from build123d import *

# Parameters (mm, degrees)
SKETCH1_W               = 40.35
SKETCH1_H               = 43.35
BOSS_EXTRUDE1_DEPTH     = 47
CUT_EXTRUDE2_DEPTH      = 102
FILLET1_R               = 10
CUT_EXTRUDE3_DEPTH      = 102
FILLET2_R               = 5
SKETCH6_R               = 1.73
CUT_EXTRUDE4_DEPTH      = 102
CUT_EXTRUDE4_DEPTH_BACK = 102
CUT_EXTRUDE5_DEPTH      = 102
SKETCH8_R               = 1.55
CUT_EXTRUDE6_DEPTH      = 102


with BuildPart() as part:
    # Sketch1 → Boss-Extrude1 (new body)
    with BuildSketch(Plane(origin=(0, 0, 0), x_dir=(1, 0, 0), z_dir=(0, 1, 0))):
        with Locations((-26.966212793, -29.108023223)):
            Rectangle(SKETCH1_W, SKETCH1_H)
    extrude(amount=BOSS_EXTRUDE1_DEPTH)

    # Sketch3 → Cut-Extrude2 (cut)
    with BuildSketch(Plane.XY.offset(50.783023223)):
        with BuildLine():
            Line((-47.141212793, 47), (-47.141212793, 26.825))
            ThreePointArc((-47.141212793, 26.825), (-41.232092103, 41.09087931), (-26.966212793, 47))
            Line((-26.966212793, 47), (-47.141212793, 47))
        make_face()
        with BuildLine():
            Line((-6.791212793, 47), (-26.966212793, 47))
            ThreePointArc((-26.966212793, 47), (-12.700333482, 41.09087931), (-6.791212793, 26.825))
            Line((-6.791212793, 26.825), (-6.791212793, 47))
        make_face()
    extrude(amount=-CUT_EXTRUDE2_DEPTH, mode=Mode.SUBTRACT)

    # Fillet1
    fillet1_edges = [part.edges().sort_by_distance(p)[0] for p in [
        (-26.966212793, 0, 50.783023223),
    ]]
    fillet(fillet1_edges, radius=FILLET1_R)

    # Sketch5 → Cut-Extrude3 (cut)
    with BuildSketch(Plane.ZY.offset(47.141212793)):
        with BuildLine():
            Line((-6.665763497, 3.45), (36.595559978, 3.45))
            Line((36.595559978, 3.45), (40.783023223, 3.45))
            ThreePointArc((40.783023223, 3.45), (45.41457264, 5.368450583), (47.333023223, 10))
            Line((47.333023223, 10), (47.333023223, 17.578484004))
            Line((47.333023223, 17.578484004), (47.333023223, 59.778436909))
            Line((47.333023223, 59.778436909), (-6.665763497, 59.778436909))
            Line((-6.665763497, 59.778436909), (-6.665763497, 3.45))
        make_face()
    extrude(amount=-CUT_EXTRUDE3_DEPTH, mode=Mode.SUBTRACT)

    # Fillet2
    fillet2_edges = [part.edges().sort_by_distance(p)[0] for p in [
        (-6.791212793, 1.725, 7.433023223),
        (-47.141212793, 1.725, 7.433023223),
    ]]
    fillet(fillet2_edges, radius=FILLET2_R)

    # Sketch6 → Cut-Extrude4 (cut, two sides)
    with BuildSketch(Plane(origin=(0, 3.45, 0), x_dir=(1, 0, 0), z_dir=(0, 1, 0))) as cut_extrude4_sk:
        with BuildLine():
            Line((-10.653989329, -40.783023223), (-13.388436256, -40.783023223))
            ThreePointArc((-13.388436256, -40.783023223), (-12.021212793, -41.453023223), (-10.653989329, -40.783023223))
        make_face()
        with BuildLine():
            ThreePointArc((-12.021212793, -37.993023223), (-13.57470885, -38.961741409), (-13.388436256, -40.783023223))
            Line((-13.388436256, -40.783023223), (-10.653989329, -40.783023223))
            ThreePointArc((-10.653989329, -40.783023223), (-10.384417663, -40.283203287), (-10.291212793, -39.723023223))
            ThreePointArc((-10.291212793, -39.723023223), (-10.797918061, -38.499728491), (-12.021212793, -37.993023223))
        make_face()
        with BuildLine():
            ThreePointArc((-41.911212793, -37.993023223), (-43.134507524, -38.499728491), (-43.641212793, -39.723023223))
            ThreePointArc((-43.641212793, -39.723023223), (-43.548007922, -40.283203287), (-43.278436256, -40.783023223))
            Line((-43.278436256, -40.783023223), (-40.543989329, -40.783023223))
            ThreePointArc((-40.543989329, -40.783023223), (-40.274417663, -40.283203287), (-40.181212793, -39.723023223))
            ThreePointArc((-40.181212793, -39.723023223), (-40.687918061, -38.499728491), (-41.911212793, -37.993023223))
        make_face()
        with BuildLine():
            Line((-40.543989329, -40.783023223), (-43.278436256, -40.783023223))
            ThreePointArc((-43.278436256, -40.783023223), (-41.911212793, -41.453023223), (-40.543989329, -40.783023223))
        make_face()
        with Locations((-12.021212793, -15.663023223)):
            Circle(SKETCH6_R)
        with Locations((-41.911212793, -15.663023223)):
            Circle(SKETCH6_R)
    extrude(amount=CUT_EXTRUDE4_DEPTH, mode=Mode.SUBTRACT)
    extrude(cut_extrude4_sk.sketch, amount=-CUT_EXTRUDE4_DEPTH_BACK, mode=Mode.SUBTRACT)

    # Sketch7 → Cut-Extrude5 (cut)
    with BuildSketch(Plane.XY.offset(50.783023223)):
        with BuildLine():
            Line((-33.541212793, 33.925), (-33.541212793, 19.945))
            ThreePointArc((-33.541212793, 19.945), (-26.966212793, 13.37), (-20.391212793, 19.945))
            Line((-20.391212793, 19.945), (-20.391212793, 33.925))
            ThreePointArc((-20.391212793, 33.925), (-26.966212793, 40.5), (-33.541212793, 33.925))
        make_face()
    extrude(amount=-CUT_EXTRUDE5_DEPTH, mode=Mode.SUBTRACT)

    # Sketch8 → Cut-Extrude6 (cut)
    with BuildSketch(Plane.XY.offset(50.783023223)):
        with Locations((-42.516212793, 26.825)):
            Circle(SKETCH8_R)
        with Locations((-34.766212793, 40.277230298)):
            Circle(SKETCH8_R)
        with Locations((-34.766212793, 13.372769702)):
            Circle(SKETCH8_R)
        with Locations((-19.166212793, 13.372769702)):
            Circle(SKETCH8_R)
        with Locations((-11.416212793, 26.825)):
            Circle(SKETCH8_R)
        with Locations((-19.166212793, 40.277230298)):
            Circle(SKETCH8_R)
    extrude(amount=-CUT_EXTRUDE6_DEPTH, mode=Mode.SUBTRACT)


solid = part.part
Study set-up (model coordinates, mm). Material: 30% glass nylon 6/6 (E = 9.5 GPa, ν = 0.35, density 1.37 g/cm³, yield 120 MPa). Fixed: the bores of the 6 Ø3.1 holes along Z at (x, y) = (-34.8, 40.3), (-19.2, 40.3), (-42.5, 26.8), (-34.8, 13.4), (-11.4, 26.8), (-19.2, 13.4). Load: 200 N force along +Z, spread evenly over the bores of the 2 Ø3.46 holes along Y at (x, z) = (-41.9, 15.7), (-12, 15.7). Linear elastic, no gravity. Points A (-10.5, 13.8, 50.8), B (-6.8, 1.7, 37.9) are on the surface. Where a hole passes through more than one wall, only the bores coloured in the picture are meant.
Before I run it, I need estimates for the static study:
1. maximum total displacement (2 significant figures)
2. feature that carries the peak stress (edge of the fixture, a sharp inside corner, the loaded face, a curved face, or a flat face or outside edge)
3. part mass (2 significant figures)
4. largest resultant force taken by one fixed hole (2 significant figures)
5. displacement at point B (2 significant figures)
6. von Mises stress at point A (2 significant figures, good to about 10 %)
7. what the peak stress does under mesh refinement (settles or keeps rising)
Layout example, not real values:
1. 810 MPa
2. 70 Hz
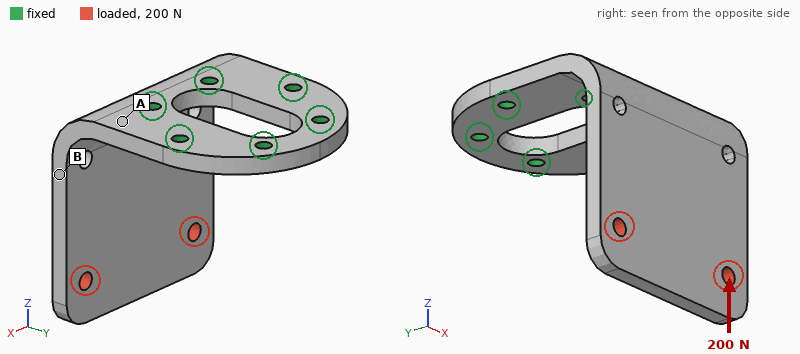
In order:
1. 0.51 mm
2. edge of the fixture
3. 13 g
4. 120 N
5. 0.16 mm
6. 11 MPa
7. keeps rising
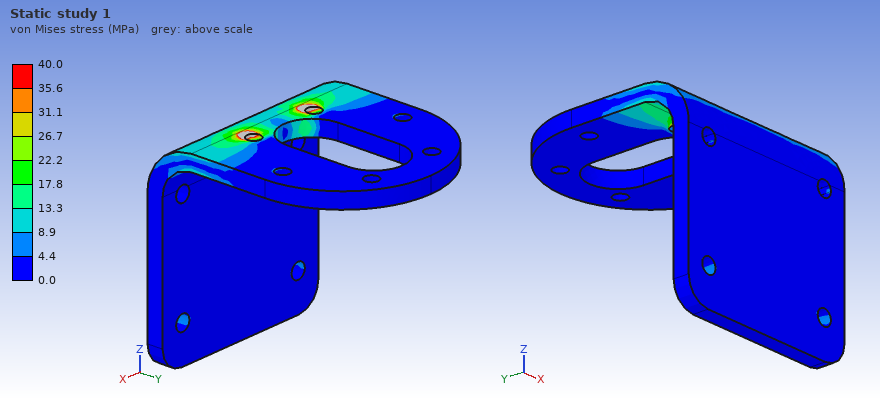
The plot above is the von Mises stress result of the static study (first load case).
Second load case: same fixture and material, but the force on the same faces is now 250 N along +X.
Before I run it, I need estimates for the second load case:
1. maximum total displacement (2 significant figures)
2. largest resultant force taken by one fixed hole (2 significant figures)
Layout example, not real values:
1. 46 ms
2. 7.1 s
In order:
1. 0.83 mm
2. 460 N
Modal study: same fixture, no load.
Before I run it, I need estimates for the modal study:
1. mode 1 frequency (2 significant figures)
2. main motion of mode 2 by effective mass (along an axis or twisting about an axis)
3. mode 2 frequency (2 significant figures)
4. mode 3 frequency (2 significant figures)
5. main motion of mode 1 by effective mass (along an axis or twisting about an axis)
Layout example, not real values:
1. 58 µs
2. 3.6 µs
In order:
1. 640 Hz
2. along X
3. 1400 Hz
4. 2300 Hz
5. along Y
